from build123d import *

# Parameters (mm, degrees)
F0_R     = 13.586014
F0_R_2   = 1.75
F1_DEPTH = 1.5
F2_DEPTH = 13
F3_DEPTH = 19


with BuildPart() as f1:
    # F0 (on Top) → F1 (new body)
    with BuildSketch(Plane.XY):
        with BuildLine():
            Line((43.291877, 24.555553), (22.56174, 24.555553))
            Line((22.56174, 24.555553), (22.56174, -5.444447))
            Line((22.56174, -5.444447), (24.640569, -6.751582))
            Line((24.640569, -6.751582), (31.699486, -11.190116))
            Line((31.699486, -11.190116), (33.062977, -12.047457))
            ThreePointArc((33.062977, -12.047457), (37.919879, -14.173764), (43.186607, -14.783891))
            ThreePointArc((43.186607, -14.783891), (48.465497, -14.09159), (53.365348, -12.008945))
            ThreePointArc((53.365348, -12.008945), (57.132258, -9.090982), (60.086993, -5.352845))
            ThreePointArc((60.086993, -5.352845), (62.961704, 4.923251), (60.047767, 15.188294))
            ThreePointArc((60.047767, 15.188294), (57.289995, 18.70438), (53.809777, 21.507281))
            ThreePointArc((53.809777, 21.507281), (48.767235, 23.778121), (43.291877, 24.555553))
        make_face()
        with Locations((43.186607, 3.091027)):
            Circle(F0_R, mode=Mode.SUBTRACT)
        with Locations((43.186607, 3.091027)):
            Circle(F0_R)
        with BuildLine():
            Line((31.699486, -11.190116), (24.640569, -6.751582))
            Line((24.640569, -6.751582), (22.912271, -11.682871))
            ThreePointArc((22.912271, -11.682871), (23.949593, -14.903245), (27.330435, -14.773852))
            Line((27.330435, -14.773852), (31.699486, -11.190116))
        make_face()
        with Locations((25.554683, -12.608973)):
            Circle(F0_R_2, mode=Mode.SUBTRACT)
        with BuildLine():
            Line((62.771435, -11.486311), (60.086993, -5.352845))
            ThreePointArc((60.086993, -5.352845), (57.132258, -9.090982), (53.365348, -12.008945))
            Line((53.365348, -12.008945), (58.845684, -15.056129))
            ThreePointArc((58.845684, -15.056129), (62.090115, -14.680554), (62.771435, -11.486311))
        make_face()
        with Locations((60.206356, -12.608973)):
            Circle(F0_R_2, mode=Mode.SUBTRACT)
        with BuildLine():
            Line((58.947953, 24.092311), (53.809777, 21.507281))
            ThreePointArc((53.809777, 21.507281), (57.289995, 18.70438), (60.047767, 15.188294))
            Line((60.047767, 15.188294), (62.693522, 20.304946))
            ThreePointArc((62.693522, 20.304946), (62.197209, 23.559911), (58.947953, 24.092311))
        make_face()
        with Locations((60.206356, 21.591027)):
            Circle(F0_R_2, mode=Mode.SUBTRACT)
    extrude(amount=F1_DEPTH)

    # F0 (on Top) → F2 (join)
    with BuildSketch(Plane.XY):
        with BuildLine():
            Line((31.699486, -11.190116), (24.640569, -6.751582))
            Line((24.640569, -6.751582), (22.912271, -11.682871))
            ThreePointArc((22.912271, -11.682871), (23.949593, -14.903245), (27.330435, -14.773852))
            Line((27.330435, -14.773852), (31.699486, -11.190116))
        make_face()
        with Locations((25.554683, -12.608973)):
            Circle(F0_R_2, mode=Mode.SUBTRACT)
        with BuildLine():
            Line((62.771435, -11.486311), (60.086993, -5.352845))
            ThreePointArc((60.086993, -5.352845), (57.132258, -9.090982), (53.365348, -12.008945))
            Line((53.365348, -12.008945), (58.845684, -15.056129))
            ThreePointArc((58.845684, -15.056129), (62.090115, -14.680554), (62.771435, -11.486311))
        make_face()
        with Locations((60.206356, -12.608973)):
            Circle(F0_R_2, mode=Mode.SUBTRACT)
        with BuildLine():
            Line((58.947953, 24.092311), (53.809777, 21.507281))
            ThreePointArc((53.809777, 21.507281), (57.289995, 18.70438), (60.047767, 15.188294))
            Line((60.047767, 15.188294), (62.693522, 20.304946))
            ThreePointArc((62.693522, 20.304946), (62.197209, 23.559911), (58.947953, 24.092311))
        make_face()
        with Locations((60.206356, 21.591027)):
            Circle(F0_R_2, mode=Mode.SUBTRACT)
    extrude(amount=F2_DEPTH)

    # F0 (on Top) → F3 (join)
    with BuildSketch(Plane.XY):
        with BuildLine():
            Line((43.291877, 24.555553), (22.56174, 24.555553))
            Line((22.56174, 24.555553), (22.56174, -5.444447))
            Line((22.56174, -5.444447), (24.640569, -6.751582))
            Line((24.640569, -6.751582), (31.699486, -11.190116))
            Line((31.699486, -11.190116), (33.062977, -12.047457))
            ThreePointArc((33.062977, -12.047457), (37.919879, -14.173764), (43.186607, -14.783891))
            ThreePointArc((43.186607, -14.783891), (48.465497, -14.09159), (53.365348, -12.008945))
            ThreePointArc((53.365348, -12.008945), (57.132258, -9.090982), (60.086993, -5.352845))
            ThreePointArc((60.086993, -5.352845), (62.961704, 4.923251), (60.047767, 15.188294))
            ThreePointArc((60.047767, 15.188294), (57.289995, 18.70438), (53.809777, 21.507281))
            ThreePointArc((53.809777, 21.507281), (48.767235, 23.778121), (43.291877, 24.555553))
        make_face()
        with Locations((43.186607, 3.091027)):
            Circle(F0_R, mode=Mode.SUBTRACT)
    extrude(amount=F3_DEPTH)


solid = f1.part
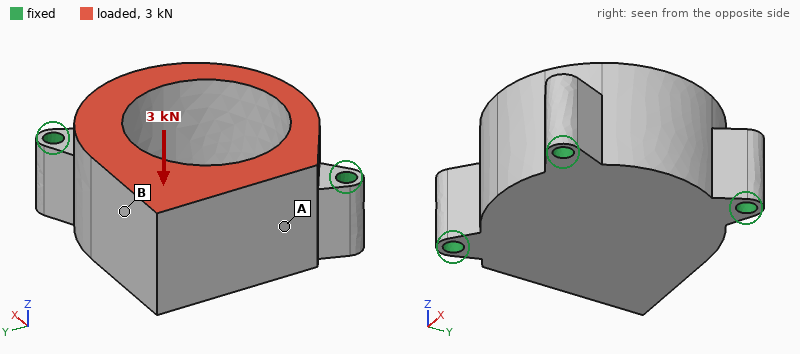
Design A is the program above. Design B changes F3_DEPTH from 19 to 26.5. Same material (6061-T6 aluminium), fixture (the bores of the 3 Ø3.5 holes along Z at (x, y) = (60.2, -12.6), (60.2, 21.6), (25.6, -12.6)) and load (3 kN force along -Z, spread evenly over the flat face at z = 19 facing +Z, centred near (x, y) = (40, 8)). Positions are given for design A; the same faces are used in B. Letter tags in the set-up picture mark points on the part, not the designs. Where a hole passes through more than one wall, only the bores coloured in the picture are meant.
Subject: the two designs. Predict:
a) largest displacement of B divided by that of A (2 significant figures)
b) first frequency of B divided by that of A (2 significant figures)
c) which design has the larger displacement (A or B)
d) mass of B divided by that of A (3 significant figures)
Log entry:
0.84
0.87
A
1.34
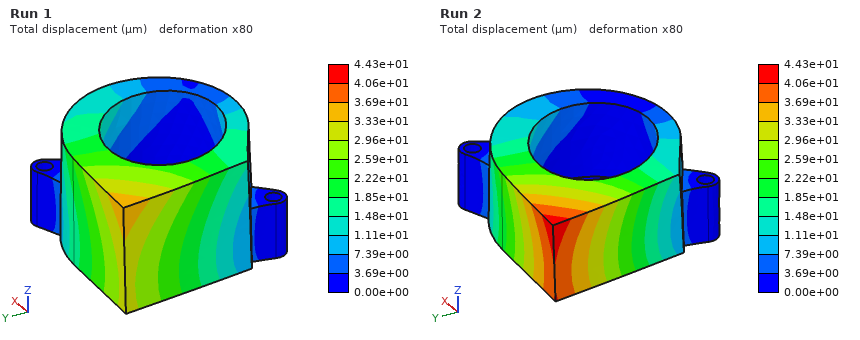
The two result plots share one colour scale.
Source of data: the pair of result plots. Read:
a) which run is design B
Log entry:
Run 1
